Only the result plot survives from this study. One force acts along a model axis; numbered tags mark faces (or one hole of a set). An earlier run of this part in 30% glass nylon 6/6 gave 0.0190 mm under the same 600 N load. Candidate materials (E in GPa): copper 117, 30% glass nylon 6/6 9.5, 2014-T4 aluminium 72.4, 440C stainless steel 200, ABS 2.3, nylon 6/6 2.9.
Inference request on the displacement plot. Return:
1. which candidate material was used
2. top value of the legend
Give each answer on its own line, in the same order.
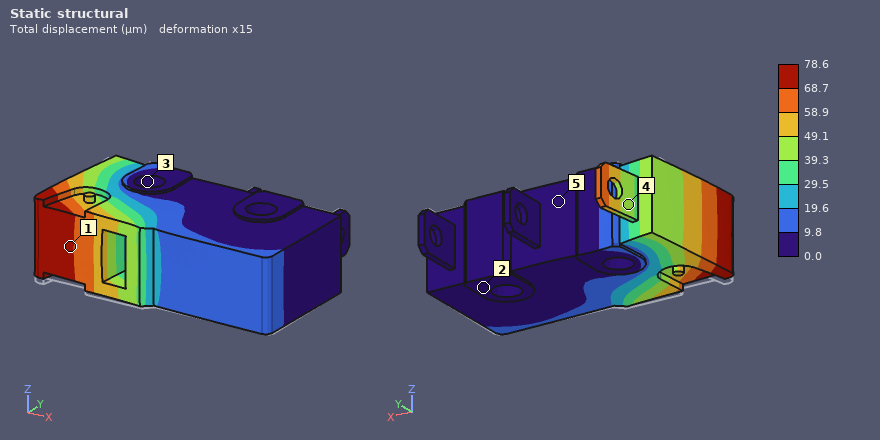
ABS
78.6 µm
